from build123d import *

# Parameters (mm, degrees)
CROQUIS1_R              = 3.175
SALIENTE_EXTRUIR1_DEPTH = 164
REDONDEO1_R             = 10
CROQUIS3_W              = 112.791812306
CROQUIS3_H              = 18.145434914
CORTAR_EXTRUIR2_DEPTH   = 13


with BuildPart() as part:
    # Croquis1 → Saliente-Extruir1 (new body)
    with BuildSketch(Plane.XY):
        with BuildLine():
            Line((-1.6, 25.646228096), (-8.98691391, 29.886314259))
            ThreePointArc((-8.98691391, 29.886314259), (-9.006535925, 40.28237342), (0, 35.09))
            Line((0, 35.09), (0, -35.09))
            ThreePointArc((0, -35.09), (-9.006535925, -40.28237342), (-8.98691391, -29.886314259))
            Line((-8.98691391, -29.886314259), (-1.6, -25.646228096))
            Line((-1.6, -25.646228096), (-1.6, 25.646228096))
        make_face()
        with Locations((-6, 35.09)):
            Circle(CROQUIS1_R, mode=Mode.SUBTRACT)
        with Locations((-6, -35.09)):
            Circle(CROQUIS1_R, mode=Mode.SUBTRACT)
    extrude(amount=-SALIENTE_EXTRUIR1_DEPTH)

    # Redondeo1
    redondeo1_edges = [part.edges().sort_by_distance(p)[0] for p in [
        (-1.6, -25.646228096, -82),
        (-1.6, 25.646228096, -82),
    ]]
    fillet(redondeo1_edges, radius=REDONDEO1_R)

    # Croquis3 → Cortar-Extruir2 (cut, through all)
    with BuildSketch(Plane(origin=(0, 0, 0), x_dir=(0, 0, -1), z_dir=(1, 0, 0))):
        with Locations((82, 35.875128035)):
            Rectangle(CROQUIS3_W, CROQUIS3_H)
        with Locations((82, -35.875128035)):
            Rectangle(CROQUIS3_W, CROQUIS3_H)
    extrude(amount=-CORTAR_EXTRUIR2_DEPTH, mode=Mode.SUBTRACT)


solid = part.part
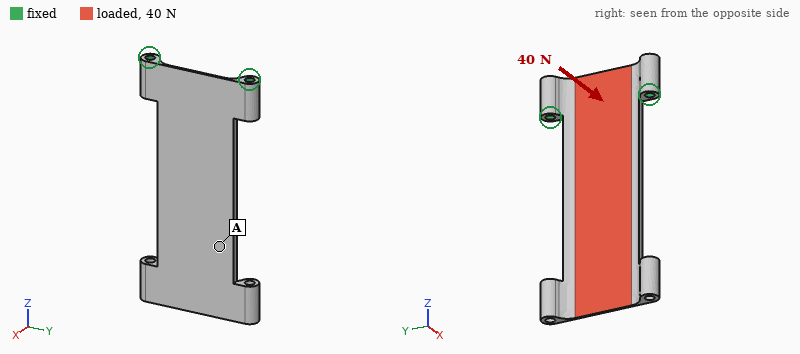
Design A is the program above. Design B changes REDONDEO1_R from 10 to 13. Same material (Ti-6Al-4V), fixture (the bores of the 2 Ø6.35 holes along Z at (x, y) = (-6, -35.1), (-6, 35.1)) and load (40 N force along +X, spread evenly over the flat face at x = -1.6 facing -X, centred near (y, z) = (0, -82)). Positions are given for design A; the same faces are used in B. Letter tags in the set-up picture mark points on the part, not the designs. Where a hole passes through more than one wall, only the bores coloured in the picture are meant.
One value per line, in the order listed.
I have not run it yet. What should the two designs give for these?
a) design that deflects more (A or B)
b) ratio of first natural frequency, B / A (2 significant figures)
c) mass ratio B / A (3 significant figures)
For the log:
A
1.2
1.04
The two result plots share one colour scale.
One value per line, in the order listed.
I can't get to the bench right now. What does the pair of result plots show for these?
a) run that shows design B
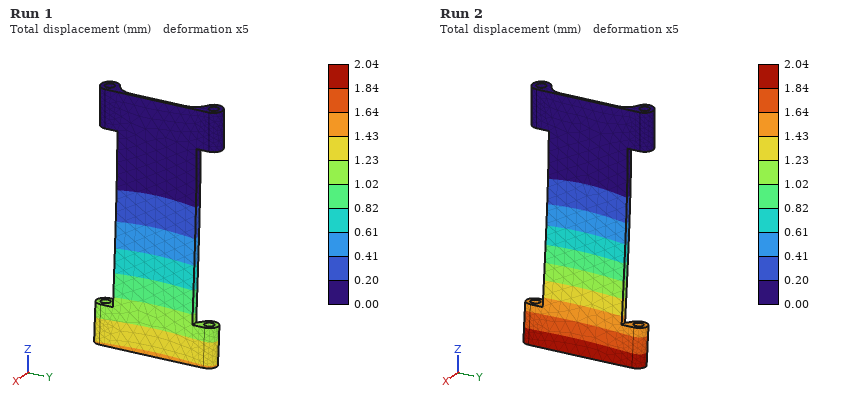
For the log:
Run 1
